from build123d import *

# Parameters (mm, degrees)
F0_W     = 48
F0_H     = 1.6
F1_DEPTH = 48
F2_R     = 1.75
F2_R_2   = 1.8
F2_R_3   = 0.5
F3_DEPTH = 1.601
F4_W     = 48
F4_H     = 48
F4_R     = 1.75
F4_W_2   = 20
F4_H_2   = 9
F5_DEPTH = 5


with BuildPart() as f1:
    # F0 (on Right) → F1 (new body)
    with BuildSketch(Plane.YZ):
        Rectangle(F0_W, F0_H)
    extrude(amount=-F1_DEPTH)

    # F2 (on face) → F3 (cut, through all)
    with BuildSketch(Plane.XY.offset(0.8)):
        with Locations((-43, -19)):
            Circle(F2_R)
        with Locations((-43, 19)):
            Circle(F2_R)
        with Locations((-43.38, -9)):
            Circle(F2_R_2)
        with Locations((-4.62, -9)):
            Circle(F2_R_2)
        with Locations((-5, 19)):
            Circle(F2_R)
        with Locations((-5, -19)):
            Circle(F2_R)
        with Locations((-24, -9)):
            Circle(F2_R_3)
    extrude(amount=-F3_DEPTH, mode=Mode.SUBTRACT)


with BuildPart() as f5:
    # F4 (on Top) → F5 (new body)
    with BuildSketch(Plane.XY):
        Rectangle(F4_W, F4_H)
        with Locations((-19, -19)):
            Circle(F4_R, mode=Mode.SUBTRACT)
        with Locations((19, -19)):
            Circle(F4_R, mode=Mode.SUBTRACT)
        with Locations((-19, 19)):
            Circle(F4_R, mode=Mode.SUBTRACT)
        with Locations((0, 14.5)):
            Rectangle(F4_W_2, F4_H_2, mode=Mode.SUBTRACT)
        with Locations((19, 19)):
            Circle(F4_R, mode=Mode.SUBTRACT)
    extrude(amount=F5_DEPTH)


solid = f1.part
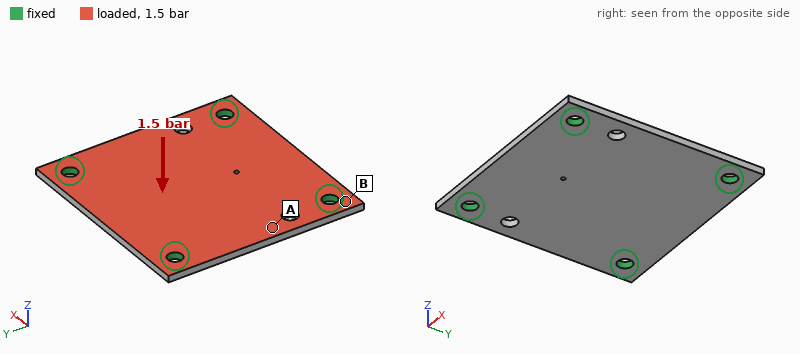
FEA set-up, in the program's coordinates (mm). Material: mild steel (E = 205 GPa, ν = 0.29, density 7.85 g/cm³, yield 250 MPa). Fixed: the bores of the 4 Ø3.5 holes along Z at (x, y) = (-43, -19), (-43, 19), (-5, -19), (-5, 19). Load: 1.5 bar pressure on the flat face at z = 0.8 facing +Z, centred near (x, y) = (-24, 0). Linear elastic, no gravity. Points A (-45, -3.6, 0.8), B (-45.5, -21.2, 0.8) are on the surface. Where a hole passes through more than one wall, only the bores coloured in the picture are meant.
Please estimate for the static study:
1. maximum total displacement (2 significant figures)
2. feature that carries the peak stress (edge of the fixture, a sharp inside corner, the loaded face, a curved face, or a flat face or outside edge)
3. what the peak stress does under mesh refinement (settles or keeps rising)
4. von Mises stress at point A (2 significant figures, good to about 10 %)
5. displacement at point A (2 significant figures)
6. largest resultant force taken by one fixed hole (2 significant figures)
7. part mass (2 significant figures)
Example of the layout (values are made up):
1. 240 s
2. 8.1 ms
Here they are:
1. 25 µm
2. edge of the fixture
3. keeps rising
4. 20 MPa
5. 11 µm
6. 85 N
7. 28 g
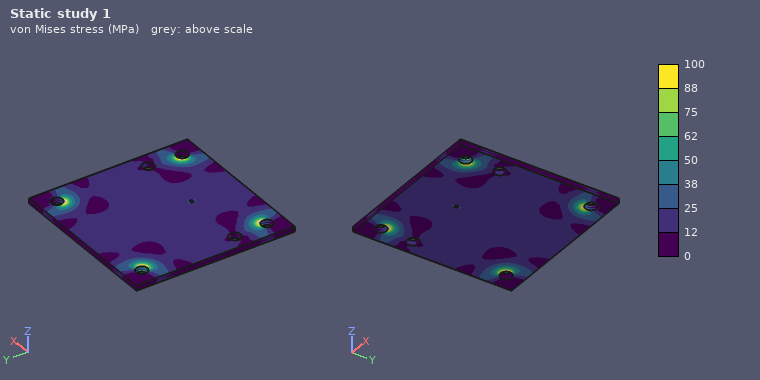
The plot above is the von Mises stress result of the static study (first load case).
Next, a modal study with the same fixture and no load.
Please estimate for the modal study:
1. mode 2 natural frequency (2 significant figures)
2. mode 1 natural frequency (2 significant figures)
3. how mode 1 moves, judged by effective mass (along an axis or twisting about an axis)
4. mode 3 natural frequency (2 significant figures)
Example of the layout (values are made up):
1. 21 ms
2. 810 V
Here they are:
1. 6900 Hz
2. 4200 Hz
3. along Z
4. 6900 Hz
